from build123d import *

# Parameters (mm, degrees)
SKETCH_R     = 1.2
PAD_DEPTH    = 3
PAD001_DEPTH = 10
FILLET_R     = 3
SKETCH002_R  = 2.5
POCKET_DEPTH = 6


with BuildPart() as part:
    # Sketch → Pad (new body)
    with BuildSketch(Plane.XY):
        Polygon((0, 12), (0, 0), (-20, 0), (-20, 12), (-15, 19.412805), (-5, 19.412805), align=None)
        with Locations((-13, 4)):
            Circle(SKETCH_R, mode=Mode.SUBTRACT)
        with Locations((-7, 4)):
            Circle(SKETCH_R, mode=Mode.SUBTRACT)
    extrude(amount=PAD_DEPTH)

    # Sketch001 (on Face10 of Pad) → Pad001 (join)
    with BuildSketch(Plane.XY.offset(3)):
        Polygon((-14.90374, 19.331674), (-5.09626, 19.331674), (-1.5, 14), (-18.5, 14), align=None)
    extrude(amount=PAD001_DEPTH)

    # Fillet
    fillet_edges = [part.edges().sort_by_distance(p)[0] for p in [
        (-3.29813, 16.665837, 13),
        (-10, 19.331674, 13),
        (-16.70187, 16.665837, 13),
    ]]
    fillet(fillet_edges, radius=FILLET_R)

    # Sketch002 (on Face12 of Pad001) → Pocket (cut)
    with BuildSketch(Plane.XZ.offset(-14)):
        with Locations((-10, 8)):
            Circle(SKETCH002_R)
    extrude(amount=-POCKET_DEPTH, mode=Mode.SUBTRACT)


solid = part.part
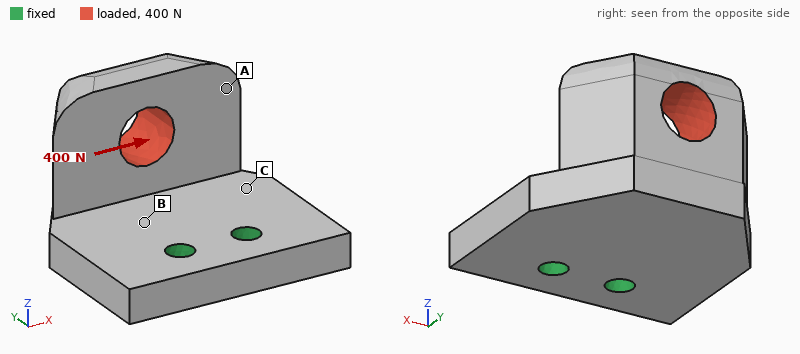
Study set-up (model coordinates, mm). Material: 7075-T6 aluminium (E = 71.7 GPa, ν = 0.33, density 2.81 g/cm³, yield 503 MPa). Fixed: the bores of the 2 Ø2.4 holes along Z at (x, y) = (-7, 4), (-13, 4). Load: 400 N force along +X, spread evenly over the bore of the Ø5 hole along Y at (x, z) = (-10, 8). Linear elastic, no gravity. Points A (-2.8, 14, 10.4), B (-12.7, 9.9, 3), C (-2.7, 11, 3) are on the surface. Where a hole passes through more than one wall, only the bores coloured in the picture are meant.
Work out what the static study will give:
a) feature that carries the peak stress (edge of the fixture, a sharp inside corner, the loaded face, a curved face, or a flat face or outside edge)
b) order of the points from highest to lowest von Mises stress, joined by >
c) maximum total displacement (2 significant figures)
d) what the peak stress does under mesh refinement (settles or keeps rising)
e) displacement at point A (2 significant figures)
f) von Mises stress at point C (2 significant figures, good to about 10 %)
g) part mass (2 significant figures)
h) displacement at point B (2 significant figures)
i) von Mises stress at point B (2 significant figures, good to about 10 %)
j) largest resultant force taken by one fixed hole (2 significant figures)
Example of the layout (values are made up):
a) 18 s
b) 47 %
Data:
a) edge of the fixture
b) B > C > A
c) 61 µm
d) keeps rising
e) 54 µm
f) 45 MPa
g) 4.5 g
h) 9.4 µm
i) 70 MPa
j) 670 N
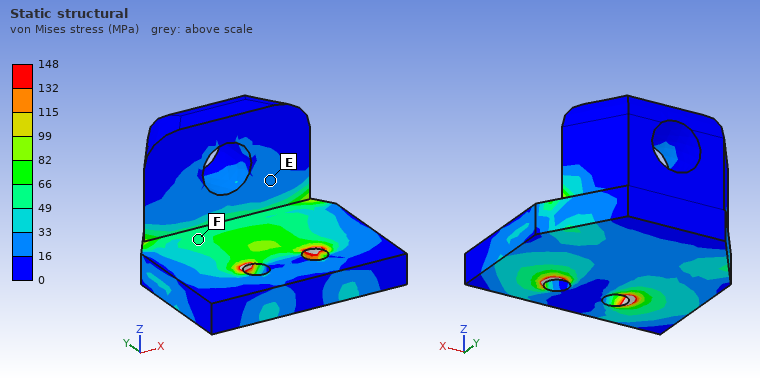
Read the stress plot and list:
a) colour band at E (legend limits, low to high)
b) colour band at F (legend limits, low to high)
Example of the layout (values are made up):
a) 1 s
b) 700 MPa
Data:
a) 16 to 33 MPa
b) 49 to 66 MPa
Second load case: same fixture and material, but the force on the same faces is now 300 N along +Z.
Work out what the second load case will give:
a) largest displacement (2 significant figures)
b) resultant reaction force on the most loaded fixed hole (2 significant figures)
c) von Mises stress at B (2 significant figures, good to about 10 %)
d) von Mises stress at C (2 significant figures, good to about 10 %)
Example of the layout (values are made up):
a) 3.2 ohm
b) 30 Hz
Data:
a) 0.11 mm
b) 150 N
c) 67 MPa
d) 53 MPa
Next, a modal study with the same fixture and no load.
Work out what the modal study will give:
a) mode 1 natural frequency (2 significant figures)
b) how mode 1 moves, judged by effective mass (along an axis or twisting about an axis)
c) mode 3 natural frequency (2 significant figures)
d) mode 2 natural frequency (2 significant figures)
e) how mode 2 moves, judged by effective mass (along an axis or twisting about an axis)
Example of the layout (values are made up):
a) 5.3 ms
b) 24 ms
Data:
a) 5800 Hz
b) along Z
c) 19 kHz
d) 11 kHz
e) along X
